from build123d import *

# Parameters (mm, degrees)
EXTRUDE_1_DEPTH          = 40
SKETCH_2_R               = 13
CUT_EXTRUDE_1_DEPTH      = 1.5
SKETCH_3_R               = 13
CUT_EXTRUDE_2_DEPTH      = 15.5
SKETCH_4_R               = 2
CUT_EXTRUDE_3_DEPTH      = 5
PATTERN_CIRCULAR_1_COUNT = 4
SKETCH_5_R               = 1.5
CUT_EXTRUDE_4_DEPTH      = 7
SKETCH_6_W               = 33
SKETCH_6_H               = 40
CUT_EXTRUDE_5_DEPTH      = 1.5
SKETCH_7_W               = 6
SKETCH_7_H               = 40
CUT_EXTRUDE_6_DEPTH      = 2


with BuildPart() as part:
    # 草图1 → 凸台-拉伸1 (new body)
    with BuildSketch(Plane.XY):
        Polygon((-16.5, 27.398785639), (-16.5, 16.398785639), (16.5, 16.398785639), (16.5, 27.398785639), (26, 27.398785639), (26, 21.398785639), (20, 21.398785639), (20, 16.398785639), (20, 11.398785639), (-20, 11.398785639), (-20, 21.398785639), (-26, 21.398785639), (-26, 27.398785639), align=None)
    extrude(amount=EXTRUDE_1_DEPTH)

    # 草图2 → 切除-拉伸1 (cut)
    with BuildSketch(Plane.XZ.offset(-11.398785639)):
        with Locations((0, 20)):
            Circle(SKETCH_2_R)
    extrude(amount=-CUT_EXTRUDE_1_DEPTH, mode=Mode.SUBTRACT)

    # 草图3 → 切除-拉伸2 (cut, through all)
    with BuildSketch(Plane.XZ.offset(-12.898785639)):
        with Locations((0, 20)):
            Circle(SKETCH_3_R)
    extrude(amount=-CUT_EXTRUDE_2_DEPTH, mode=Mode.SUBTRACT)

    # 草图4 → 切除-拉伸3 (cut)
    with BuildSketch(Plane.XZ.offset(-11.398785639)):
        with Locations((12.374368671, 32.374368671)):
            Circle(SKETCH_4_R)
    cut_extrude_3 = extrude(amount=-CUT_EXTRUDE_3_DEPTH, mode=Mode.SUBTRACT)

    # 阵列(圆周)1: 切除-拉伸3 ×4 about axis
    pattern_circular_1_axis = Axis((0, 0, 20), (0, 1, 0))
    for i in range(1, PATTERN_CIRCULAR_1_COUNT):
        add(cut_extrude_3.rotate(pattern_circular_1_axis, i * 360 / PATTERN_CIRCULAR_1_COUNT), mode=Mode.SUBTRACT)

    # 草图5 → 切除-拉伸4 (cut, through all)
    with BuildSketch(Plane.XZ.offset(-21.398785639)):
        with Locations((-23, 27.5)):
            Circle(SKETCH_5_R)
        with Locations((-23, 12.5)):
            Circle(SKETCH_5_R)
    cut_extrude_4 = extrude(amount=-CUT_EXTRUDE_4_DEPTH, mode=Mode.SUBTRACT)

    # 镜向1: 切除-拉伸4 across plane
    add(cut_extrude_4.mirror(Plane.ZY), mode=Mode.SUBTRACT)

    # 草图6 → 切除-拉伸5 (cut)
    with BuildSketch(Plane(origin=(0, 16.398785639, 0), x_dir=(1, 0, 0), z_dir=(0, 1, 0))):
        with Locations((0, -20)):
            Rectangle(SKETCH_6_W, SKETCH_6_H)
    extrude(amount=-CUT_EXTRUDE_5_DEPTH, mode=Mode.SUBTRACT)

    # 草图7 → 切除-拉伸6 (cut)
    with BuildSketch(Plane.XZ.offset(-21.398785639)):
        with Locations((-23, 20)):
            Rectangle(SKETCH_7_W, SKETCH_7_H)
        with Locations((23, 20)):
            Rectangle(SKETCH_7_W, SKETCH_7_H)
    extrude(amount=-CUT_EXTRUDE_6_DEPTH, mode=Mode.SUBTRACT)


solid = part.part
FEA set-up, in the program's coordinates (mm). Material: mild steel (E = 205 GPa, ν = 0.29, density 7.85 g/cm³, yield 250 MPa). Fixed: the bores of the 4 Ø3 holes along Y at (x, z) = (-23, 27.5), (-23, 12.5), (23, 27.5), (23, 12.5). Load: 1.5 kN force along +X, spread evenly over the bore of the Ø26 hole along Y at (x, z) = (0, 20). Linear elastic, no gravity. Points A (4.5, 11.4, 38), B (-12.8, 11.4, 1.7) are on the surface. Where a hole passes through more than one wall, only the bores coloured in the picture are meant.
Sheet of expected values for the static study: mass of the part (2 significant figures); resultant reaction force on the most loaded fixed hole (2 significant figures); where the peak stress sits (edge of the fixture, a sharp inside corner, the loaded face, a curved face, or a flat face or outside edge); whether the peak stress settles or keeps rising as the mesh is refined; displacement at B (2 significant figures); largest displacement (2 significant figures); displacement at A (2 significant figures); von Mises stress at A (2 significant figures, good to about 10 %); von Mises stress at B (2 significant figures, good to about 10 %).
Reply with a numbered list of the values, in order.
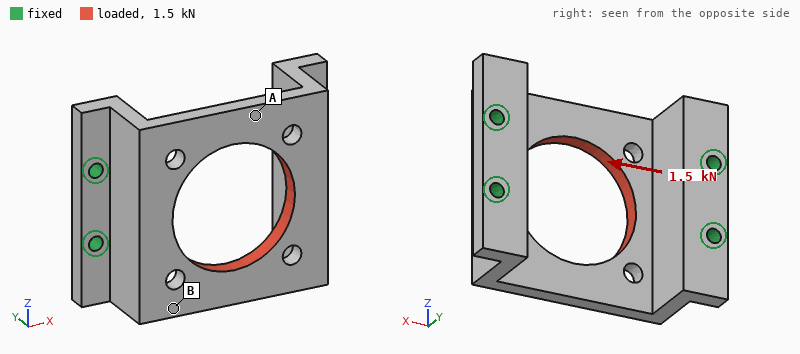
1. 70 g
2. 400 N
3. edge of the fixture
4. keeps rising
5. 17 µm
6. 20 µm
7. 15 µm
8. 24 MPa
9. 52 MPa
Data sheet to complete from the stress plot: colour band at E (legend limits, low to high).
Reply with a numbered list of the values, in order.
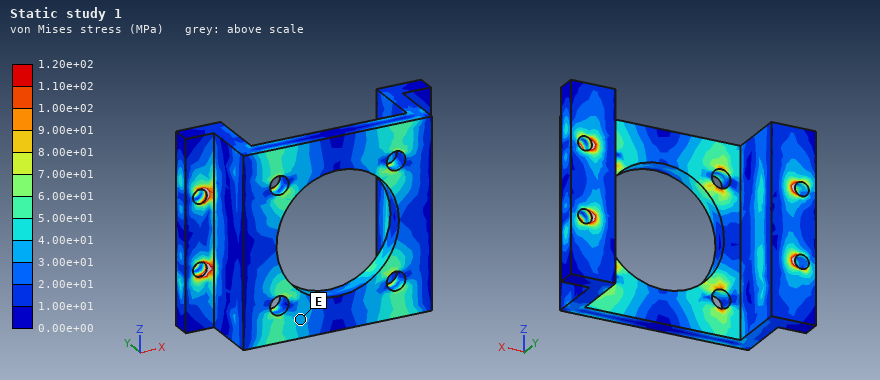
1. 3.00e+01 to 4.00e+01 MPa
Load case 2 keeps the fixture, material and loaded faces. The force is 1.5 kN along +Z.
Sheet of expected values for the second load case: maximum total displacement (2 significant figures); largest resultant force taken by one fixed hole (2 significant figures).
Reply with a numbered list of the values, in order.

1. 7.5 µm
2. 670 N
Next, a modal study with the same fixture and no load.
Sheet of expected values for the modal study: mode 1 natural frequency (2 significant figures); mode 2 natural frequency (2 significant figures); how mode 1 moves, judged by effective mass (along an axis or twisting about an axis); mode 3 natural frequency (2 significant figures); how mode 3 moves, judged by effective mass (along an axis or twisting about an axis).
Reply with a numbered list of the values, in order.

1. 8100 Hz
2. 11 kHz
3. along X
4. 12 kHz
5. twisting about Y
